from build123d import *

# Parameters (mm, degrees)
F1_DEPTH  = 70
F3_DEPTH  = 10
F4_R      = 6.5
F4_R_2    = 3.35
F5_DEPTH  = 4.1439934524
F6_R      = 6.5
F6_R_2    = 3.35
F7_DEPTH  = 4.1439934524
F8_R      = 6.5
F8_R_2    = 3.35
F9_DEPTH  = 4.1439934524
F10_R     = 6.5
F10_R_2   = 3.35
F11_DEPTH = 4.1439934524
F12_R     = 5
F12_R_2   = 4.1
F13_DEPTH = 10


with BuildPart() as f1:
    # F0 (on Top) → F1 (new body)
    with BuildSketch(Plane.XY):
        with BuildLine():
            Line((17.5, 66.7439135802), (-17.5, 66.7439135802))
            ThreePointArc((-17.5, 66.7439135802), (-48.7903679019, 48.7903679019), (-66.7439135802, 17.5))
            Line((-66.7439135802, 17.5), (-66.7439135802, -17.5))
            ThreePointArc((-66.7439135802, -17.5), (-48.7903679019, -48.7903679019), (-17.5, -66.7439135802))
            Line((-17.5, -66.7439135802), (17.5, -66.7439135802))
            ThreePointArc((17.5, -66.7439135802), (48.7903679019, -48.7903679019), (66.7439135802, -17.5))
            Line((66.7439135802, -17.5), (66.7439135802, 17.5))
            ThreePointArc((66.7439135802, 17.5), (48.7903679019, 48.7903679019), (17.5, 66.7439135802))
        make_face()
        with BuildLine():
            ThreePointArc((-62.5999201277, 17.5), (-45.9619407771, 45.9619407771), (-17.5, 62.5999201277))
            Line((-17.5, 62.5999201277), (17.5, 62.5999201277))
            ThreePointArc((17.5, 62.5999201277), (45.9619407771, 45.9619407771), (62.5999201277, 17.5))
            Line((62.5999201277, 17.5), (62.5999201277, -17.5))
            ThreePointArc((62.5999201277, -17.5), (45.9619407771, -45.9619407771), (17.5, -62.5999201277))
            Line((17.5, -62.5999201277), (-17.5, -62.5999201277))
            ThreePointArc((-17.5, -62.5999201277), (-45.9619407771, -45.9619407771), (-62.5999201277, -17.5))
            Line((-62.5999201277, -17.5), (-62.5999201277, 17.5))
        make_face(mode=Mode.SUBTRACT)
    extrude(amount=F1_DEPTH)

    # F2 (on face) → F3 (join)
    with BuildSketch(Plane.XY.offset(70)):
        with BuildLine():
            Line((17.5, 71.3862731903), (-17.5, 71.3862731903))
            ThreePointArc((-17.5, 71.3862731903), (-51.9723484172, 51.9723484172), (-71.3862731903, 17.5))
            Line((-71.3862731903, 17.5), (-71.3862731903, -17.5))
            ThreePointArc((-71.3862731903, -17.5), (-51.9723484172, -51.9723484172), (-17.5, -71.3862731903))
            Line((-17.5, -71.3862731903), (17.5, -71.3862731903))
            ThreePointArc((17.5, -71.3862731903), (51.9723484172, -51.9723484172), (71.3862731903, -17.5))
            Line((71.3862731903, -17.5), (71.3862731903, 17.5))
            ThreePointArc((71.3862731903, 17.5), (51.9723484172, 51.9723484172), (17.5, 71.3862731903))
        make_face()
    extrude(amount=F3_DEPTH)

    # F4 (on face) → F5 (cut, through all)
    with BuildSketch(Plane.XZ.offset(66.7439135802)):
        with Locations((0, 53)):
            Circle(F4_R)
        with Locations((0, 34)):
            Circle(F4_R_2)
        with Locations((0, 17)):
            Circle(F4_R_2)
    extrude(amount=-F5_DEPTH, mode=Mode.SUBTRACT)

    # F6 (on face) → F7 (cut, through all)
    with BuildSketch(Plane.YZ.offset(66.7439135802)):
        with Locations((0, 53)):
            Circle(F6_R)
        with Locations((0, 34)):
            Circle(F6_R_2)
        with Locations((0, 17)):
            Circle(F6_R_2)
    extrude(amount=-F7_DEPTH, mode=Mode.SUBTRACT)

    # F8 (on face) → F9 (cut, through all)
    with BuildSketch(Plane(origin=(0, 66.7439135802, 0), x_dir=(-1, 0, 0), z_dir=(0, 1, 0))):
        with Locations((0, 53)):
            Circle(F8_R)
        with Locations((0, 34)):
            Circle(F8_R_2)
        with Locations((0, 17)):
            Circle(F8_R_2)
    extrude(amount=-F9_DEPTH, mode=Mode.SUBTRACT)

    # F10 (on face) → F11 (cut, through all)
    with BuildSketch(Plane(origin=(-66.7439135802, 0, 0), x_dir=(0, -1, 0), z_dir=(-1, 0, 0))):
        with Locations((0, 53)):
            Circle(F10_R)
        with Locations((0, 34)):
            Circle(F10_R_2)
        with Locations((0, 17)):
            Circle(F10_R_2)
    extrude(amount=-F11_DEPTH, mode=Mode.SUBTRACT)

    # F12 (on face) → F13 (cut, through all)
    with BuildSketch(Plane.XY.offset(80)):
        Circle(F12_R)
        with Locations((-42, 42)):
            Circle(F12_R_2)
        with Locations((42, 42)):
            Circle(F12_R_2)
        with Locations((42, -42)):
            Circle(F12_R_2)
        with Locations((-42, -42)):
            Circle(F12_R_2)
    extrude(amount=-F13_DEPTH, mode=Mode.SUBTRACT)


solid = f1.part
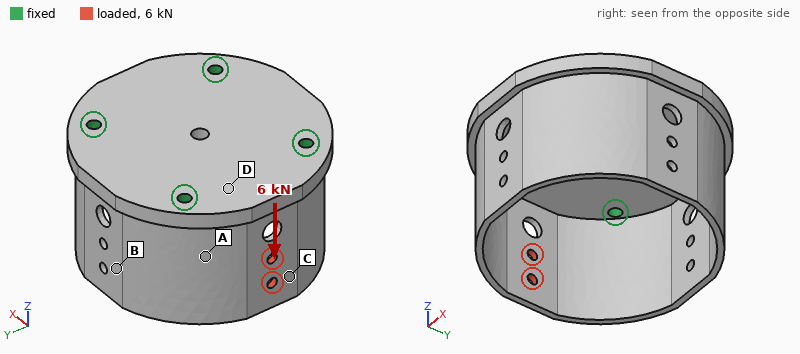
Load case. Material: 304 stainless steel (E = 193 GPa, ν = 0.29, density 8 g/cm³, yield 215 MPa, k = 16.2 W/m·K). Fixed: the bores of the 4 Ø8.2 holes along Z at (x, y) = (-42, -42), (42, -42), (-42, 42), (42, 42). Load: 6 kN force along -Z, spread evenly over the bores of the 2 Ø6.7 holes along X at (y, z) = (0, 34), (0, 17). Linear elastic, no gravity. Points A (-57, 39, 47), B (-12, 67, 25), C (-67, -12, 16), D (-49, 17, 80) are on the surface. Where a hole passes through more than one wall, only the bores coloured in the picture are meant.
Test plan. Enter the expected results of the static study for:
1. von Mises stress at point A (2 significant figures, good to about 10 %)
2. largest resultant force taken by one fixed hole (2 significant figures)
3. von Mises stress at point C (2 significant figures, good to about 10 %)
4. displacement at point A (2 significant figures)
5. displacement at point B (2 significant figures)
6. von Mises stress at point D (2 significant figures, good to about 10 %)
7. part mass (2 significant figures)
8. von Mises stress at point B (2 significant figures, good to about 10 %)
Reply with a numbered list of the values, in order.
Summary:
1. 27 MPa
2. 3.5 kN
3. 32 MPa
4. 15 µm
5. 31 µm
6. 18 MPa
7. 2.2 kg
8. 9.9 MPa
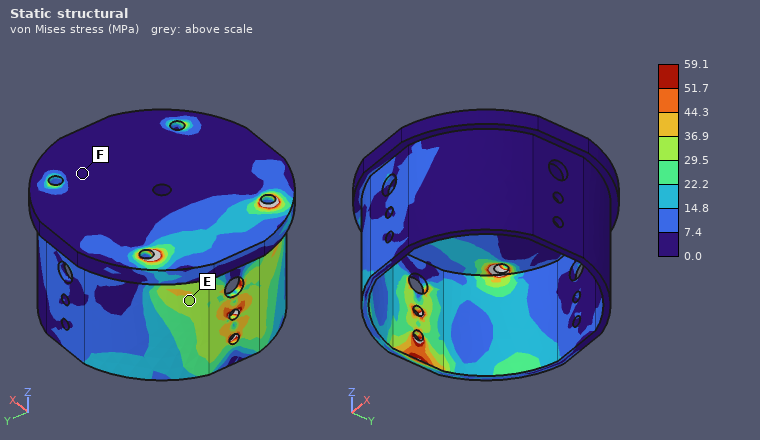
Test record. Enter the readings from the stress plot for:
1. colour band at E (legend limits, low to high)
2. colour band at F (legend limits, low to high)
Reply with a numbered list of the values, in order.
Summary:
1. 29.5 to 36.9 MPa
2. 0.0 to 7.4 MPa
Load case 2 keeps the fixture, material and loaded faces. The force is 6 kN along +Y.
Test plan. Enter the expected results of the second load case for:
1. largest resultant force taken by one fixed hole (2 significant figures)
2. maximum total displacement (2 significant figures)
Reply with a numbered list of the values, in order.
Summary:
1. 5.0 kN
2. 62 µm
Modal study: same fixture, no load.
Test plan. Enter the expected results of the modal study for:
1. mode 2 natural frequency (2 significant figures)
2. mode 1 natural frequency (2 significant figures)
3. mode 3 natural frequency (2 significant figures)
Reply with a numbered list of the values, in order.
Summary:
1. 2200 Hz
2. 1600 Hz
3. 2200 Hz
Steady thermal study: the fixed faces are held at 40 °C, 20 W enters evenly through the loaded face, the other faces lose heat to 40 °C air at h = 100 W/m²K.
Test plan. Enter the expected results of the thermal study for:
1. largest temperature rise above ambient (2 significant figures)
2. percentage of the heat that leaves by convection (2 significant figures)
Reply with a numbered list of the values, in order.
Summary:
1. 68 K
2. 97 %
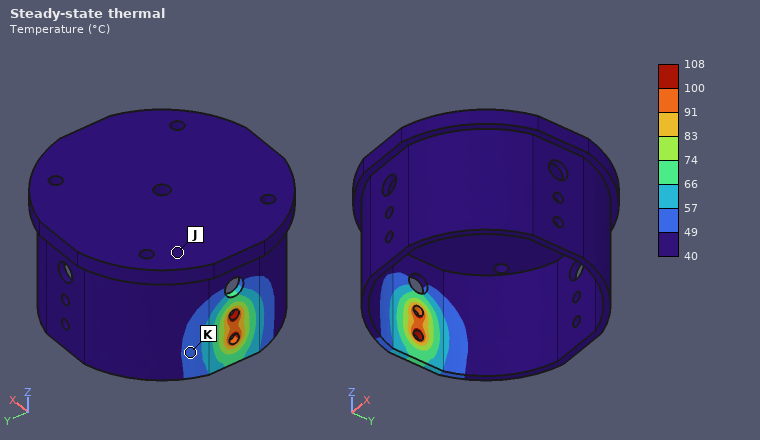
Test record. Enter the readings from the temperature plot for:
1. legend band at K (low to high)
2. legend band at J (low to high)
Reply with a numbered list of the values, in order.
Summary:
1. 49 to 57 °C
2. 40 to 49 °C
